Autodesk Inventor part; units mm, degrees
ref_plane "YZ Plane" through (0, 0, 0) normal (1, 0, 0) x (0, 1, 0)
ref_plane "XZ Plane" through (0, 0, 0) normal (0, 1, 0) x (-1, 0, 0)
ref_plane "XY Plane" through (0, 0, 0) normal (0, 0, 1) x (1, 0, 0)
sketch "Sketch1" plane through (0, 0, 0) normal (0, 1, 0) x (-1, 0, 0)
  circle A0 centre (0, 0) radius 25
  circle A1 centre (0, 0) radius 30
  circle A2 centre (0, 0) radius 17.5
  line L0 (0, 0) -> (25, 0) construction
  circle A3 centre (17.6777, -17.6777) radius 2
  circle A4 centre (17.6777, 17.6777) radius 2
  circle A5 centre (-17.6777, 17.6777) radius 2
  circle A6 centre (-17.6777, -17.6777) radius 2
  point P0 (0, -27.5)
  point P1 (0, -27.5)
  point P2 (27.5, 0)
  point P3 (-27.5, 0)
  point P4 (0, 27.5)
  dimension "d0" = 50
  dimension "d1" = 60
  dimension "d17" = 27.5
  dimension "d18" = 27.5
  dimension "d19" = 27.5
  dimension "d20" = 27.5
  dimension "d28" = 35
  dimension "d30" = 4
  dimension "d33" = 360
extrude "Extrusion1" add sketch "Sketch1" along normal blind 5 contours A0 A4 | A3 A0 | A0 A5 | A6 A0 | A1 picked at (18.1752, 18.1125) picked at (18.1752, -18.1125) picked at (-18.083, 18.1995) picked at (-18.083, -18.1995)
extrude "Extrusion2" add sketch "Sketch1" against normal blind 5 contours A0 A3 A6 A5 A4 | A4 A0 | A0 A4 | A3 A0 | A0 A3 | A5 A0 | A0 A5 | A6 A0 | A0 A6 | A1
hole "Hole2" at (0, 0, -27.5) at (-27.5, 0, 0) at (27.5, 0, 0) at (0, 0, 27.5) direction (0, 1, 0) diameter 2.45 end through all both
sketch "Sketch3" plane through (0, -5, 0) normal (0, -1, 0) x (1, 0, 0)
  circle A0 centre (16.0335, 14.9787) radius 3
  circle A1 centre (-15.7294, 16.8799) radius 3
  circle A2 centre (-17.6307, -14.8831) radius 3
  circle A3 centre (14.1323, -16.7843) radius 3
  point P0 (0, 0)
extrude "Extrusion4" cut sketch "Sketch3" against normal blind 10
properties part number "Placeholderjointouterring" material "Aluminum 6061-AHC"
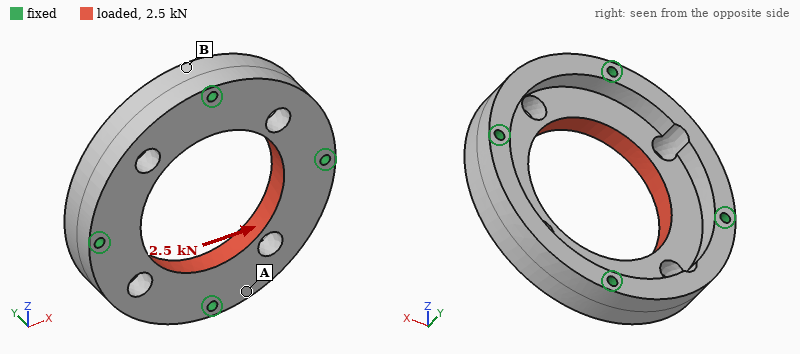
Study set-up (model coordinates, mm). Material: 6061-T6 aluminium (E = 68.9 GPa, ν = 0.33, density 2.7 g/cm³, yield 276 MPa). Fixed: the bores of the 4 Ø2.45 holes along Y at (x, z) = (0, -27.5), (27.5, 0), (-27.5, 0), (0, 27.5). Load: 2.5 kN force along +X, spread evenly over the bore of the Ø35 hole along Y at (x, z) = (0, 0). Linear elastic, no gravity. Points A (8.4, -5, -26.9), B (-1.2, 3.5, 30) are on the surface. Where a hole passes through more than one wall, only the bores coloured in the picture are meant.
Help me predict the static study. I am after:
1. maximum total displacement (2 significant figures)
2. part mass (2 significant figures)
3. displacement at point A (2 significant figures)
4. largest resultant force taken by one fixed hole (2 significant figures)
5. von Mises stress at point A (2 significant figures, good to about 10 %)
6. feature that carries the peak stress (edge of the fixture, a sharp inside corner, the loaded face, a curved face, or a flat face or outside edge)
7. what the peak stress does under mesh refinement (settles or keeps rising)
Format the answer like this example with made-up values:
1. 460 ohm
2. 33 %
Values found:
1. 5.0 µm
2. 35 g
3. 2.0 µm
4. 720 N
5. 7.0 MPa
6. edge of the fixture
7. keeps rising
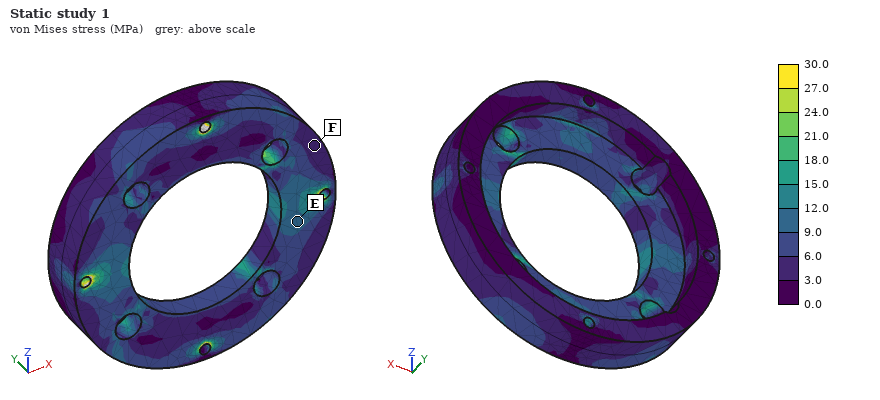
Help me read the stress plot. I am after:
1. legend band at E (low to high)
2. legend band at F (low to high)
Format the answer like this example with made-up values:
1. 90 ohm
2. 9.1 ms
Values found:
1. 9.0 to 12.0 MPa
2. 3.0 to 6.0 MPa
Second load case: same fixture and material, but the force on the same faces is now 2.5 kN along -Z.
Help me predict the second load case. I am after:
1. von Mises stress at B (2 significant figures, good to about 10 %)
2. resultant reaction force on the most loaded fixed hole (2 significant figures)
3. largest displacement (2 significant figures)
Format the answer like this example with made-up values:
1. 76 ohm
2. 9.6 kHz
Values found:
1. 5.5 MPa
2. 730 N
3. 5.0 µm
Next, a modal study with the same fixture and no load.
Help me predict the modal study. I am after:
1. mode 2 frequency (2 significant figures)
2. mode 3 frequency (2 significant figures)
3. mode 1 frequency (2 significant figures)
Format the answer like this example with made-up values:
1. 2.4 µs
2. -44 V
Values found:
1. 20 kHz
2. 20 kHz
3. 19 kHz
